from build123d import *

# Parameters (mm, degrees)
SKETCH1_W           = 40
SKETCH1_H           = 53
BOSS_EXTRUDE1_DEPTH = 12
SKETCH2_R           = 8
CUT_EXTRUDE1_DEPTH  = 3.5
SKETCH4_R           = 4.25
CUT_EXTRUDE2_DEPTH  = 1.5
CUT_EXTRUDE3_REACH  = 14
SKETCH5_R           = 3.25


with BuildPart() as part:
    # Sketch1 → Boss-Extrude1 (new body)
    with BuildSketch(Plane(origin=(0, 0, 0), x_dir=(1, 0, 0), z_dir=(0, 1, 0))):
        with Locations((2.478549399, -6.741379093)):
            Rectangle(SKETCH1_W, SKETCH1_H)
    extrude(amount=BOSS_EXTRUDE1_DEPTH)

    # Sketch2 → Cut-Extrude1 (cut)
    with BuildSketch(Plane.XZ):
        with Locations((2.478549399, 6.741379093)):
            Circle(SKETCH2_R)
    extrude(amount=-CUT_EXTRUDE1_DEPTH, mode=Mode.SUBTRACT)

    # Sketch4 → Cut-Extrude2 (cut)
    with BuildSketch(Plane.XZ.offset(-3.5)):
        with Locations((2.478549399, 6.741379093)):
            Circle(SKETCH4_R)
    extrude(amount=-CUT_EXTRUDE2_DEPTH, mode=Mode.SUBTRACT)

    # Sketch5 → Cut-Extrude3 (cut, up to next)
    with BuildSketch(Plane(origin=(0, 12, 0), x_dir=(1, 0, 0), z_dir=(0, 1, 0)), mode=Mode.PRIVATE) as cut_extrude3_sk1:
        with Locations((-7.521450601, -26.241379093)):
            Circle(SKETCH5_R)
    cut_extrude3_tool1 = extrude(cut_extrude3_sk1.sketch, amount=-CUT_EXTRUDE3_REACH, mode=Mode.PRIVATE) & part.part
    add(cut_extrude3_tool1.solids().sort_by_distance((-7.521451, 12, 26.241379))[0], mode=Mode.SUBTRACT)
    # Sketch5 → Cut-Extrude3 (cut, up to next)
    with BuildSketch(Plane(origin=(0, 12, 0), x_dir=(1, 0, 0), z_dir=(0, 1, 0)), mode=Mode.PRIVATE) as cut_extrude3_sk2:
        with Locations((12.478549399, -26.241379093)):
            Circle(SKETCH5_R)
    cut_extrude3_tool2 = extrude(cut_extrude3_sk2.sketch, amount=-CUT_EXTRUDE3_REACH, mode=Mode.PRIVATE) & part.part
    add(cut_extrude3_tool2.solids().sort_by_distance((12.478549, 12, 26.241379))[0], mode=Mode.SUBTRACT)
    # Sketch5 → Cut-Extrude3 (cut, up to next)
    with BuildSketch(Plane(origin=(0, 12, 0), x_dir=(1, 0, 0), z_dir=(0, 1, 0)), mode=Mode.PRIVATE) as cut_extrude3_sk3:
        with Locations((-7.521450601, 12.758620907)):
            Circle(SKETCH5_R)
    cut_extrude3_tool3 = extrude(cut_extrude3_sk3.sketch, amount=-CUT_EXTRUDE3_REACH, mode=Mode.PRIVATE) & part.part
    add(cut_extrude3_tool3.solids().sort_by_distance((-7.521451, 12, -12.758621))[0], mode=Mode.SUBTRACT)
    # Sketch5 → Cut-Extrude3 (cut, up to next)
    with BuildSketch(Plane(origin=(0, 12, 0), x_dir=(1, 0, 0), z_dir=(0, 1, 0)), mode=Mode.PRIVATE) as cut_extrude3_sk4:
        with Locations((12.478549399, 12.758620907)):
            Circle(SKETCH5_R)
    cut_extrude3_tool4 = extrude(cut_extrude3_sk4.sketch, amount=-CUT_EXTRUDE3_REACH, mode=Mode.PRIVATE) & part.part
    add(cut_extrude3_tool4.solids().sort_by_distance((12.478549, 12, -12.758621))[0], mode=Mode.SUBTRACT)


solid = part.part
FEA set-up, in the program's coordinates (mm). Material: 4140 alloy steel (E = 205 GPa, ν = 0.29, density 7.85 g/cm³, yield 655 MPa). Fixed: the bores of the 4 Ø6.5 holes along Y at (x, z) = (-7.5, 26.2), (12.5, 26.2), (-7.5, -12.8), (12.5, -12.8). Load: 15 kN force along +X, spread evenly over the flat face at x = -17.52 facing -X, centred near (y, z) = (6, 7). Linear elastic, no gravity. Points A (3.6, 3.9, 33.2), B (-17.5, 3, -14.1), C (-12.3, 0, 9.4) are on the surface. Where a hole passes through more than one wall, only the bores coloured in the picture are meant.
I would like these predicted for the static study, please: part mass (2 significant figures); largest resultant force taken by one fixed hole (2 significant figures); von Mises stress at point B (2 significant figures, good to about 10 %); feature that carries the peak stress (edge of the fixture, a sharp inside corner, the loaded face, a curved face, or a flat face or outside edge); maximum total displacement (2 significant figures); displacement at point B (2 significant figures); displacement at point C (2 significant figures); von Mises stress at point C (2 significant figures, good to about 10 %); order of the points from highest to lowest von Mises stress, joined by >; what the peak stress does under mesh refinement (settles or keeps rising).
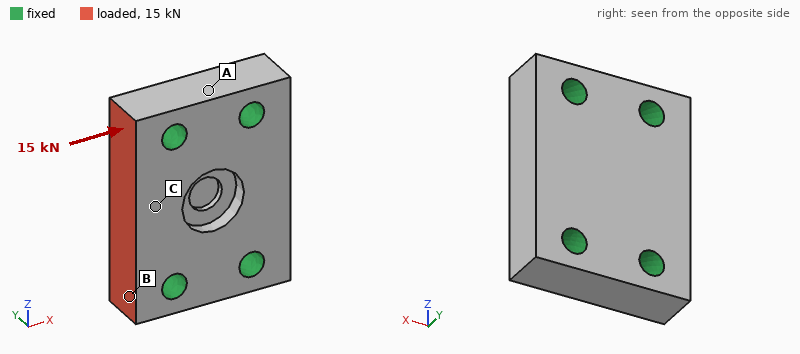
180 g
5.9 kN
31 MPa
edge of the fixture
3.5 µm
1.00 µm
2.9 µm
18 MPa
B > C > A
keeps rising
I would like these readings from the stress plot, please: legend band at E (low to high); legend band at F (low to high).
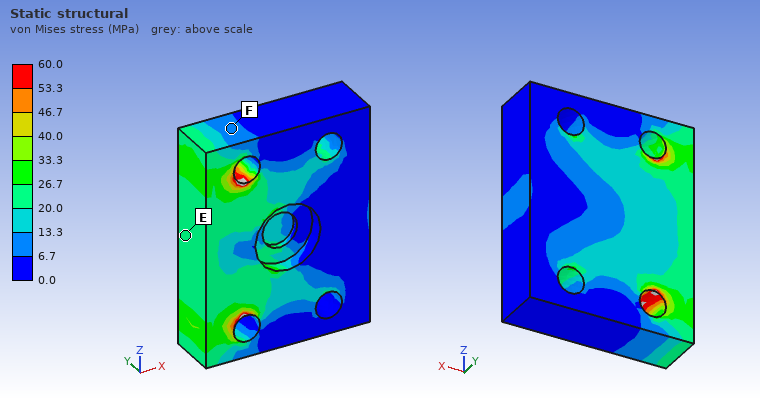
20.0 to 26.7 MPa
6.7 to 13.3 MPa
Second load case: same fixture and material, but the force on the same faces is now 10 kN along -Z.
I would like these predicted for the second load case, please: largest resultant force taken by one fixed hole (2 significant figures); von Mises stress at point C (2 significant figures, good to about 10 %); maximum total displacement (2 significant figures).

5.1 kN
24 MPa
3.9 µm
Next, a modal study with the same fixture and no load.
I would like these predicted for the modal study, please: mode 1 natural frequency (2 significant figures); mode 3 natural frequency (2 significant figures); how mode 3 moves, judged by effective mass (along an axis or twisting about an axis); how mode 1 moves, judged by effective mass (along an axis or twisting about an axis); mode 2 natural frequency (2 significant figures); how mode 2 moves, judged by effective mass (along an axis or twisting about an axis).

30 kHz
39 kHz
along X
along Y
32 kHz
twisting about Z
